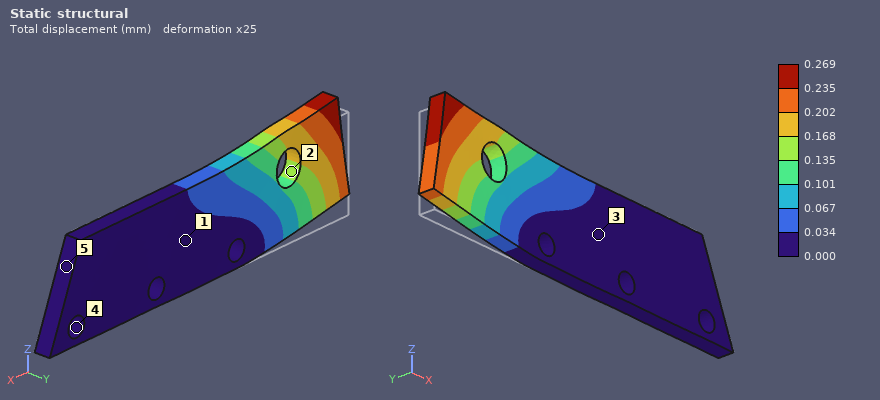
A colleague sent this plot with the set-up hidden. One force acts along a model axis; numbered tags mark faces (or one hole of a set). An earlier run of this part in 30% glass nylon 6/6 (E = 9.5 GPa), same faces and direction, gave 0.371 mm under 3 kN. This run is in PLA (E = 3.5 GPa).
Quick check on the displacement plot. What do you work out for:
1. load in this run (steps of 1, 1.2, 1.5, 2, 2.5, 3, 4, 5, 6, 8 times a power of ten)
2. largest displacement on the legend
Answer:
800 N
0.269 mm
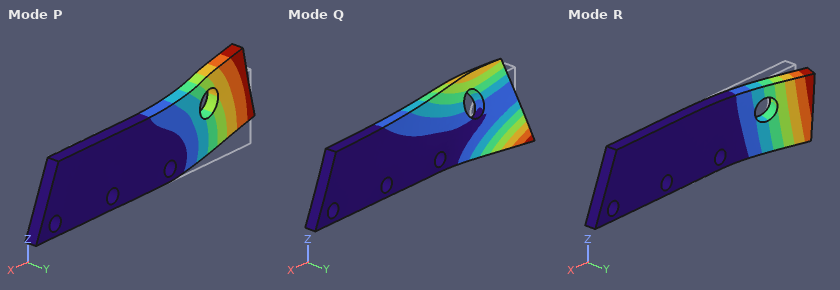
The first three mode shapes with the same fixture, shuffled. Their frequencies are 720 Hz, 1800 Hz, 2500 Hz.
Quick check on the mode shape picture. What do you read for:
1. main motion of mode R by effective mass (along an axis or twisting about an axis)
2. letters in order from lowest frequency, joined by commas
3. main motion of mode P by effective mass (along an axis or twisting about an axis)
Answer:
along Y
R, Q, P
along Z
